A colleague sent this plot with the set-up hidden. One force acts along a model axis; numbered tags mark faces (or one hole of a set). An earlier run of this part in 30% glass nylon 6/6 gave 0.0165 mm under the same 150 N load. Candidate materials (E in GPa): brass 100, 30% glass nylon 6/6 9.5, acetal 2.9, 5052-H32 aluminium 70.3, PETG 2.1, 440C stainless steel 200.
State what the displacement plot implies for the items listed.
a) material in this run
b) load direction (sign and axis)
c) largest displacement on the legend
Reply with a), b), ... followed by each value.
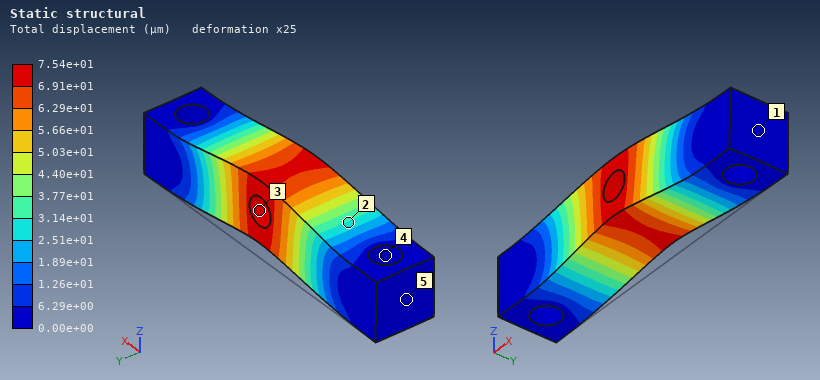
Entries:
a) PETG
b) +Z
c) 7.54e+01 µm
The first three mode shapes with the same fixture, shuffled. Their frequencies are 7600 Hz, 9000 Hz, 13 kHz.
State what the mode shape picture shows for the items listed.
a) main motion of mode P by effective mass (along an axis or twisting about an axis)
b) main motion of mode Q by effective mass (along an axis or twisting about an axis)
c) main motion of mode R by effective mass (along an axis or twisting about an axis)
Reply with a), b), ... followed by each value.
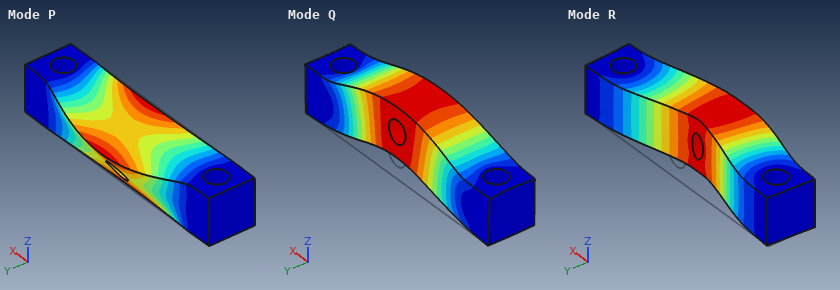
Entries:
a) twisting about X
b) along Z
c) along Y
